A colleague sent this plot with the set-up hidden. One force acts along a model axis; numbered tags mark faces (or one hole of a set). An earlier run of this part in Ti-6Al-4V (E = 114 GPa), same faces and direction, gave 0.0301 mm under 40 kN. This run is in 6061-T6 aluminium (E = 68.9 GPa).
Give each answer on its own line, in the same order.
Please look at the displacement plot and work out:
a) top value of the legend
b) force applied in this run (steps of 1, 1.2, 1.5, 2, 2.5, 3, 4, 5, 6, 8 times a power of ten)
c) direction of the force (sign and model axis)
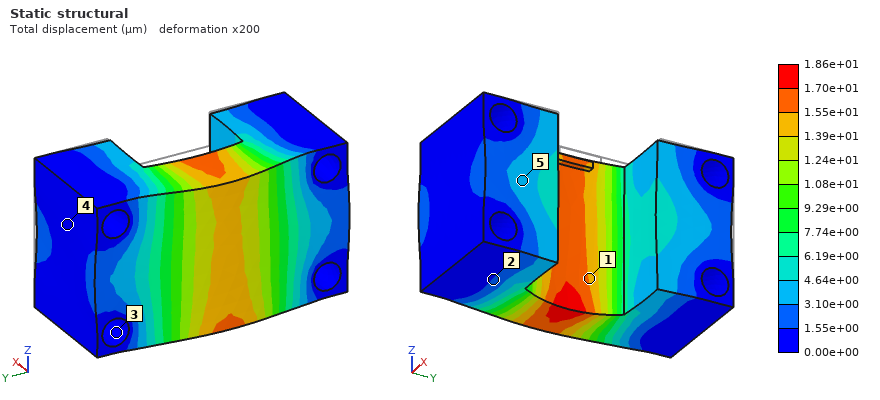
1.86e+01 µm
15 kN
-X
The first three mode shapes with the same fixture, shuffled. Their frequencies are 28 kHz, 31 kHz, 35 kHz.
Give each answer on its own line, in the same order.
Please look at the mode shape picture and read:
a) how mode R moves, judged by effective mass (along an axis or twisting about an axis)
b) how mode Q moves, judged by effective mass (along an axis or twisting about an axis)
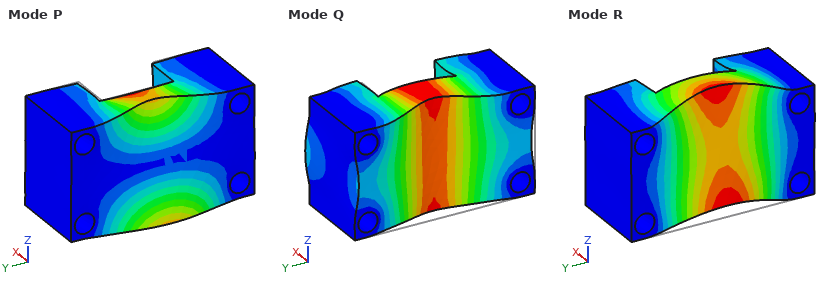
along Z
along X
